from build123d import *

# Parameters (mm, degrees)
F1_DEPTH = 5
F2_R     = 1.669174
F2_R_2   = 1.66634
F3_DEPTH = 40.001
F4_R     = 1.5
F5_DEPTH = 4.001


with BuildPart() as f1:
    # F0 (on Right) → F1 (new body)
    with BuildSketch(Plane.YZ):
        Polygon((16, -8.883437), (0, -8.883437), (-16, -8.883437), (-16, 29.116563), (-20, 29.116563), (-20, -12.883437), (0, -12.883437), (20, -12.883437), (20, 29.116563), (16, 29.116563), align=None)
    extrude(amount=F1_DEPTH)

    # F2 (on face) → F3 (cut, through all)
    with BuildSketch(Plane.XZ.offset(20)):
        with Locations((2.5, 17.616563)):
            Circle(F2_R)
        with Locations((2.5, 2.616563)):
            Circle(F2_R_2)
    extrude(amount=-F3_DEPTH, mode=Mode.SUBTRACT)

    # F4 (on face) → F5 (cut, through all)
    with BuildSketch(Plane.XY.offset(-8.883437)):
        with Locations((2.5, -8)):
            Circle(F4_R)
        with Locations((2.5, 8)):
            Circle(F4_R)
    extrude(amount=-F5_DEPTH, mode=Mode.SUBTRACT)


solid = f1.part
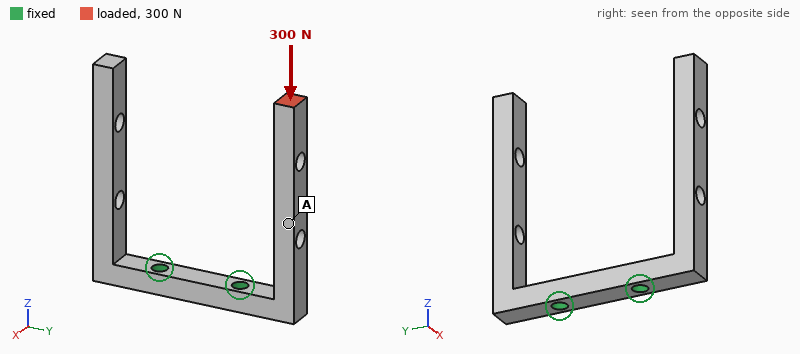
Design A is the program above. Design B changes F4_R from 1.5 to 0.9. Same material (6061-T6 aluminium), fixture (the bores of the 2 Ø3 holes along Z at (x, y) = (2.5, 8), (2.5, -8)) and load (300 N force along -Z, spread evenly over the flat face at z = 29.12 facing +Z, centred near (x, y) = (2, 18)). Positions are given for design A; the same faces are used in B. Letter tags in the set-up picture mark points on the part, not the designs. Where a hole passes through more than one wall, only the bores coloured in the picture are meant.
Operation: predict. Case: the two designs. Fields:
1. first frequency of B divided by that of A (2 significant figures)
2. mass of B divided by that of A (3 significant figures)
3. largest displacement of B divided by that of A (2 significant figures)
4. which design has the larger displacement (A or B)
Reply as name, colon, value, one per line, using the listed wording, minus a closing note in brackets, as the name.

first frequency of B divided by that of A: 0.98
mass of B divided by that of A: 1.02
largest displacement of B divided by that of A: 1.2
which design has the larger displacement: B
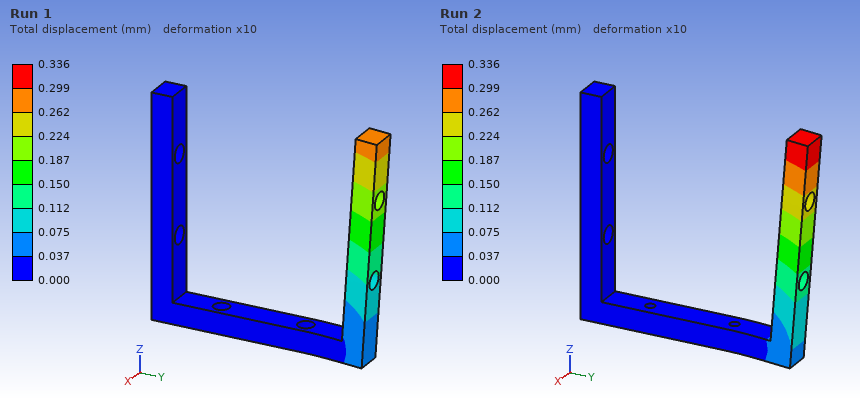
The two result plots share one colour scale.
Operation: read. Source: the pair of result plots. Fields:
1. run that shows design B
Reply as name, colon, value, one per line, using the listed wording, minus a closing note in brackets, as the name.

run that shows design B: Run 2
